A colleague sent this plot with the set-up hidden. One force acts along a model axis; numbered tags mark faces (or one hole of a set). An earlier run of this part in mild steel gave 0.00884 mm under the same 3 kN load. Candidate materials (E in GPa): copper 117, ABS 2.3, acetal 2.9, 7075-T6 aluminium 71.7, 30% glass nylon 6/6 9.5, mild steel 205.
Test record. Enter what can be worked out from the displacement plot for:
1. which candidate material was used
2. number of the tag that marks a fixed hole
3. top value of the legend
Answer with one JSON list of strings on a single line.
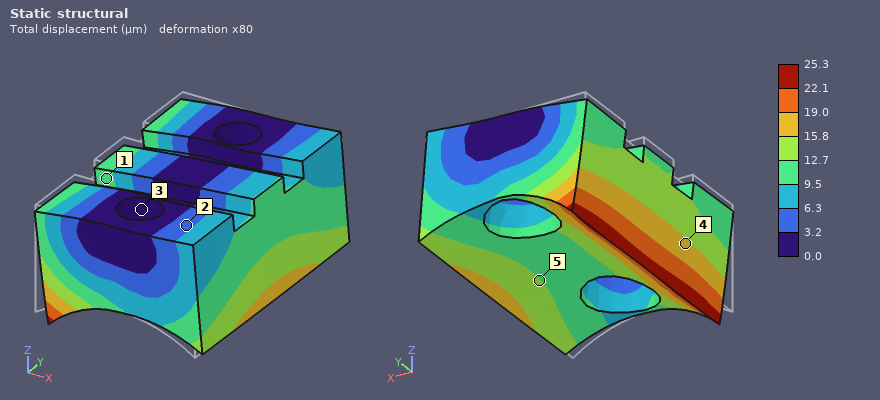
["7075-T6 aluminium", "3", "25.3 µm"]
